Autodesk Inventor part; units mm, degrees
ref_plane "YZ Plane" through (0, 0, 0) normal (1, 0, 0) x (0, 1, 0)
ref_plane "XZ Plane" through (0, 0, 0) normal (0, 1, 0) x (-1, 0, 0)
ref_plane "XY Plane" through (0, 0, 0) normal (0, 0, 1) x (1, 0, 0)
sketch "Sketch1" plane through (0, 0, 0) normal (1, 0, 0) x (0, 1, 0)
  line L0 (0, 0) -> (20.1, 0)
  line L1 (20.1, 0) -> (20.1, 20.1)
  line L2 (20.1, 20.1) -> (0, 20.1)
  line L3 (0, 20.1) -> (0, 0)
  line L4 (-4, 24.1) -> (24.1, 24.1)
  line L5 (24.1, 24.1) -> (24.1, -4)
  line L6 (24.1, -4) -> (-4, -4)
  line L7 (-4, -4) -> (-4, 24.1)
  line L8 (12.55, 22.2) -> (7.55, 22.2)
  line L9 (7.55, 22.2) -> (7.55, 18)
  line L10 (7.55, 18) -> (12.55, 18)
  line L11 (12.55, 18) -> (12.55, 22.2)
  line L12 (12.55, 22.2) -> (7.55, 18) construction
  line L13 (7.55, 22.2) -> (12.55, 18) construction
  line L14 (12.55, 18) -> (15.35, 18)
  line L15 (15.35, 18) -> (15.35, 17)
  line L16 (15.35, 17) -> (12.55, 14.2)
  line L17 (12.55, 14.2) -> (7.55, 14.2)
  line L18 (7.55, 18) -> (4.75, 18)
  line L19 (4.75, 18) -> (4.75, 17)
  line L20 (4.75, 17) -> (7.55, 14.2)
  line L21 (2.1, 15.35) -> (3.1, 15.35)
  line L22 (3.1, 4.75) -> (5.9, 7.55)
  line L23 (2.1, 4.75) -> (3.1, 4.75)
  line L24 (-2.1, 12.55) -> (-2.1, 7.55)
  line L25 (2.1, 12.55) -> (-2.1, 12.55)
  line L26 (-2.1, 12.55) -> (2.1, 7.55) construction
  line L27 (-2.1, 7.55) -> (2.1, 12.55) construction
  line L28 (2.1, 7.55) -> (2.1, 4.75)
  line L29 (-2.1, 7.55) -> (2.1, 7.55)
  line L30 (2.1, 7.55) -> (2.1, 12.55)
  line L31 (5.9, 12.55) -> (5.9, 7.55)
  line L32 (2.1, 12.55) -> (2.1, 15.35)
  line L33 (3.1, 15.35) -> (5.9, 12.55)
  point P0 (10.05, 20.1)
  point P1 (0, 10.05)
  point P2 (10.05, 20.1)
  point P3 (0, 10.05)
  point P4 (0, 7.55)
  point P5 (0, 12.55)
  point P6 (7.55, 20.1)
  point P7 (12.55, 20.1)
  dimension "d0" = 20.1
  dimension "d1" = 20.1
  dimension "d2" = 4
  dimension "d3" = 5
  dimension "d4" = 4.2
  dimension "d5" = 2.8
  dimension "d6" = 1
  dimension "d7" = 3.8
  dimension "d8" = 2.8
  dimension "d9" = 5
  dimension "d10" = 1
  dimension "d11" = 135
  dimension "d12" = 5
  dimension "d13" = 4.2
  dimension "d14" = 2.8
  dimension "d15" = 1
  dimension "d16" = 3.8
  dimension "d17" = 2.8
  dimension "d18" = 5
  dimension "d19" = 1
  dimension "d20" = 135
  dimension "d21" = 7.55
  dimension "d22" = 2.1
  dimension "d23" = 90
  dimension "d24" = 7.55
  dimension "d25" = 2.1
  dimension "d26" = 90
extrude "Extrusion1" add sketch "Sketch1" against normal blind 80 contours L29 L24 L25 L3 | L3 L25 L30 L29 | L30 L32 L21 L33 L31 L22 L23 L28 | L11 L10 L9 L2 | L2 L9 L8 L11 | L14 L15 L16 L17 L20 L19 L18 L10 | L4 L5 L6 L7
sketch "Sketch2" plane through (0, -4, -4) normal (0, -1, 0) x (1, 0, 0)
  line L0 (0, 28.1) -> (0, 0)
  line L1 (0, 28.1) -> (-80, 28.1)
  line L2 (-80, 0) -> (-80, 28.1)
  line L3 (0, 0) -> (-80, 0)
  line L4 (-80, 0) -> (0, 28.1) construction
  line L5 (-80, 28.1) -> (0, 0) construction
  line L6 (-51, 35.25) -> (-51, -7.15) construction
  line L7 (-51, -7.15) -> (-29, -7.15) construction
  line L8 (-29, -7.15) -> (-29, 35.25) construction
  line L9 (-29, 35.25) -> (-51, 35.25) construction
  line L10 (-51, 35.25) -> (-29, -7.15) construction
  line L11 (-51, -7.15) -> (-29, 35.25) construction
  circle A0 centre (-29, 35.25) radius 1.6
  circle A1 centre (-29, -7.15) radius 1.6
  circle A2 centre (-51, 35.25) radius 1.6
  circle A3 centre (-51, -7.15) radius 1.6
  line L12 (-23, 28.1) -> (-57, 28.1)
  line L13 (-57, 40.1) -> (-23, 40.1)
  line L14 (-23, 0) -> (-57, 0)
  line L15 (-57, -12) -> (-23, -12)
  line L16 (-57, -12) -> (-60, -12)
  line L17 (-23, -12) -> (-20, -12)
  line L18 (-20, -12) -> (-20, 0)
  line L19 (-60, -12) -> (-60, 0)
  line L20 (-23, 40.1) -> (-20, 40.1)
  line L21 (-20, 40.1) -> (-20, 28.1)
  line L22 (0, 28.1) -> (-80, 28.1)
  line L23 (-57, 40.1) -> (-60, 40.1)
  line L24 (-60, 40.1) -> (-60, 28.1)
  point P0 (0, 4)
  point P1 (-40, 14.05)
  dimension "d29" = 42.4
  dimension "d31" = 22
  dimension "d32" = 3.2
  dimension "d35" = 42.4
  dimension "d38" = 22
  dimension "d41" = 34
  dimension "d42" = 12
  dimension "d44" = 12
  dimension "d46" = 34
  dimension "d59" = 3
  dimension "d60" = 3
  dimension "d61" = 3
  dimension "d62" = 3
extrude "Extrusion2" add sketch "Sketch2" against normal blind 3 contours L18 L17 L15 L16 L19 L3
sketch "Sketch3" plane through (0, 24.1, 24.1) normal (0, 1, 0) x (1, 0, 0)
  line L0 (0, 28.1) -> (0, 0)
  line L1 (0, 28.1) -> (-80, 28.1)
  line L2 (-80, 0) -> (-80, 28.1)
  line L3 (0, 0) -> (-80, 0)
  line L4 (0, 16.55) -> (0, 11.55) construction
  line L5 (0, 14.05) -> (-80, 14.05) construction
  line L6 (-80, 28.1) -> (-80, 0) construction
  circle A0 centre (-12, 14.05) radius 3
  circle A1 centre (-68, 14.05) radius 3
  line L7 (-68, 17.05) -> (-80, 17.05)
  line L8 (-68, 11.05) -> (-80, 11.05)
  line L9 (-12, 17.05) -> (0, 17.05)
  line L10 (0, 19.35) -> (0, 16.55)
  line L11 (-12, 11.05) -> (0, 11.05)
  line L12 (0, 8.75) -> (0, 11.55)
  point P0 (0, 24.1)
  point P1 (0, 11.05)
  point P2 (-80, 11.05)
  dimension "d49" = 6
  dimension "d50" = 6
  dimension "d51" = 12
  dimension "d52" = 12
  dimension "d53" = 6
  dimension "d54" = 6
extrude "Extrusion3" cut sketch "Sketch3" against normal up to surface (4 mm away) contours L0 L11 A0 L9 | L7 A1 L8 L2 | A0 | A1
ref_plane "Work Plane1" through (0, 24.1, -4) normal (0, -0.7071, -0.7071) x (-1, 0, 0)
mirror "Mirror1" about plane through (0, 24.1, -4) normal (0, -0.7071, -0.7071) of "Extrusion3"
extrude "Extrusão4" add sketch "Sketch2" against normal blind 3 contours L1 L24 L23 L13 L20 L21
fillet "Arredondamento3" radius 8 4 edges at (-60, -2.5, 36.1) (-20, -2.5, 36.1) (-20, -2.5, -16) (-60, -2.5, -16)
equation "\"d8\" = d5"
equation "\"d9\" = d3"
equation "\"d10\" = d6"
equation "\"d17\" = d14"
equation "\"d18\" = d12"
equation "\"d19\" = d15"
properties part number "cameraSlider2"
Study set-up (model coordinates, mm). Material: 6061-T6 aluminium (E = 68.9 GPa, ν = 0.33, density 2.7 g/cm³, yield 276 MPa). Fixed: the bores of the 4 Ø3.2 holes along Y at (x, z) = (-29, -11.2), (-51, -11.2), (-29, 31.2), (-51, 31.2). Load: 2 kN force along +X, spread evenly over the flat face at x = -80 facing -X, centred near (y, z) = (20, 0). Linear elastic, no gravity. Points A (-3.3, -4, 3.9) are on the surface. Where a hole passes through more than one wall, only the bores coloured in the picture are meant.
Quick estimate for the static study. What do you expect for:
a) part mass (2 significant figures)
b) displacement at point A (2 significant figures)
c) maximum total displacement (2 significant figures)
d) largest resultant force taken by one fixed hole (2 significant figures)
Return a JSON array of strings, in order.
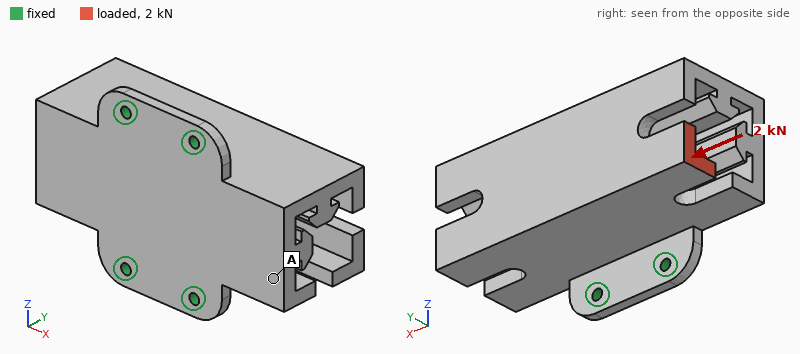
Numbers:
["110 g", "0.11 mm", "0.17 mm", "1.2 kN"]
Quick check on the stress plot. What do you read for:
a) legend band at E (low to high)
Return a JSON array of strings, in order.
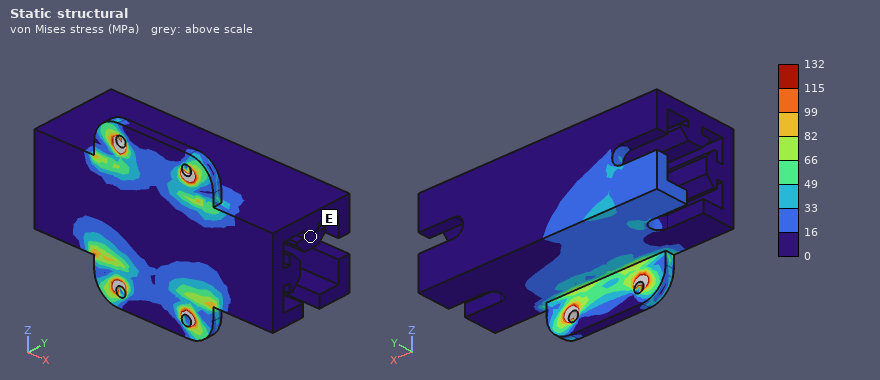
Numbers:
["0 to 16 MPa"]
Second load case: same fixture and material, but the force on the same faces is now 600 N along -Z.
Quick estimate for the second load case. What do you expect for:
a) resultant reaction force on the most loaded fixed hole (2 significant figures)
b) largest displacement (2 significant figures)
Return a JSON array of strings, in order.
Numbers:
["380 N", "0.12 mm"]
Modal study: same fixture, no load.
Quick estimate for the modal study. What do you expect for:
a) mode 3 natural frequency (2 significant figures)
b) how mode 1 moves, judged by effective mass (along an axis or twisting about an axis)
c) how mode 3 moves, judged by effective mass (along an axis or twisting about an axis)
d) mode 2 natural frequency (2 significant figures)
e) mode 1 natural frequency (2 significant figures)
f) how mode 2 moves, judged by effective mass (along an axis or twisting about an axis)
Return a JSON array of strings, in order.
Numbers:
["4900 Hz", "along X", "along Y", "3900 Hz", "2300 Hz", "along Z"]
